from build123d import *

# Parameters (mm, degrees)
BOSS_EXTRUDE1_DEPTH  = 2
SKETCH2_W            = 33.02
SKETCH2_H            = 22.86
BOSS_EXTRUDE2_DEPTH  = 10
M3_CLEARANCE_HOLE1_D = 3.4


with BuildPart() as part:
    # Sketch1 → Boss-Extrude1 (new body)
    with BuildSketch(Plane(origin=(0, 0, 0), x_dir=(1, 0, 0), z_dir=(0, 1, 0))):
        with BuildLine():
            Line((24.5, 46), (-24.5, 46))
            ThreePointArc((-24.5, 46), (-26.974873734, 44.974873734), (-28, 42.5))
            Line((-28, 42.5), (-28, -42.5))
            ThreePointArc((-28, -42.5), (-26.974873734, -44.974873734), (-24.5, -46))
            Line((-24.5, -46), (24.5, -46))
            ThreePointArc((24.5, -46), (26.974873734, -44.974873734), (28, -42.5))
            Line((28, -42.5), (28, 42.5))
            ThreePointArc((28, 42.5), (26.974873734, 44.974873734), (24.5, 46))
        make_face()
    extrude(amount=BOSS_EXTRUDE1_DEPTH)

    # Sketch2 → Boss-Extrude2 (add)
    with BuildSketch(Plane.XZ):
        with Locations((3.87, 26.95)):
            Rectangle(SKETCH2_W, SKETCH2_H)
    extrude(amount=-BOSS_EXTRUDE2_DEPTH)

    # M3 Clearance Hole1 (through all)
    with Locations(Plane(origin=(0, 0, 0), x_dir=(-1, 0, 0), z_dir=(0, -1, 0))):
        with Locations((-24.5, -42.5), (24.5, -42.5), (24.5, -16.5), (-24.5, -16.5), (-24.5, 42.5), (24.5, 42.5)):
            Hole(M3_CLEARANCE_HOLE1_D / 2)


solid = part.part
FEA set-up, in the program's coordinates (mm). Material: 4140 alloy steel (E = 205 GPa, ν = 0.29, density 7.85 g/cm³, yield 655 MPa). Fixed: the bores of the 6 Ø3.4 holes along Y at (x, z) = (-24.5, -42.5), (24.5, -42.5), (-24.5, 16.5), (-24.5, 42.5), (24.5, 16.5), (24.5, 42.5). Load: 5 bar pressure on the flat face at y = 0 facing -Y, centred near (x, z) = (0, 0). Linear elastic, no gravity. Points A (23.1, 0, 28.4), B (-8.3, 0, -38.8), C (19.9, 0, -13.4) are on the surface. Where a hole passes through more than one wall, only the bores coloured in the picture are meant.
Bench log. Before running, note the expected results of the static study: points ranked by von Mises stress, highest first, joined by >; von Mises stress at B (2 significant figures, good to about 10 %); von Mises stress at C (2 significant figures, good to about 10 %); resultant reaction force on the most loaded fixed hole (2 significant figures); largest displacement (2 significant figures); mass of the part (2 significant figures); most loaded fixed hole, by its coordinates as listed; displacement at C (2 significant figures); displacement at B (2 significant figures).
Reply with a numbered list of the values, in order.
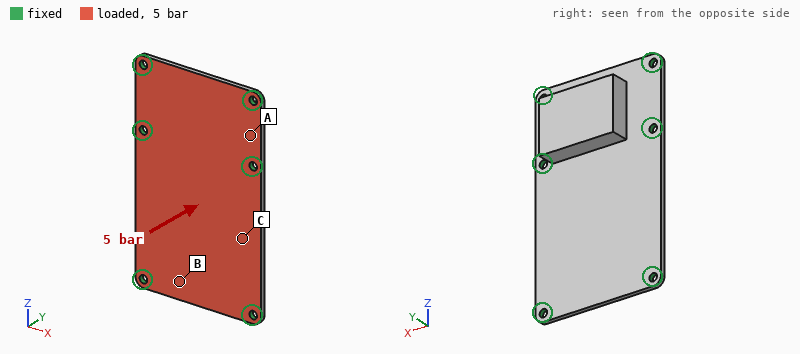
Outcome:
1. C > B > A
2. 72 MPa
3. 120 MPa
4. 930 N
5. 0.17 mm
6. 130 g
7. (24.5, 16.5)
8. 0.14 mm
9. 0.076 mm
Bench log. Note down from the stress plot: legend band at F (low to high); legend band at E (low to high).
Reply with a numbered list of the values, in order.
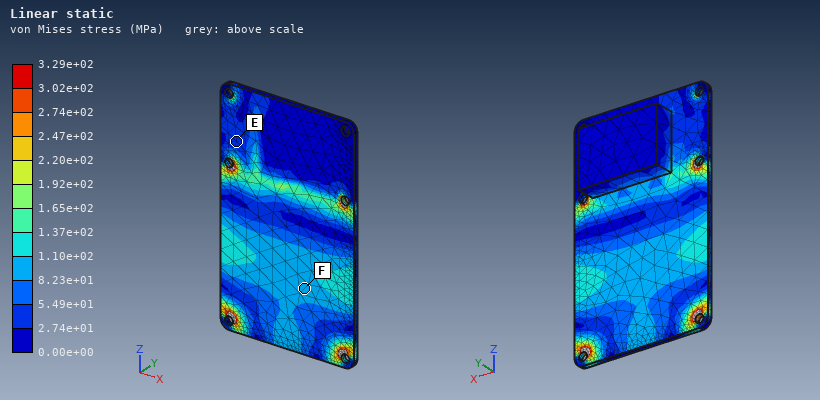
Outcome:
1. 8.23e+01 to 1.10e+02 MPa
2. 2.74e+01 to 5.49e+01 MPa
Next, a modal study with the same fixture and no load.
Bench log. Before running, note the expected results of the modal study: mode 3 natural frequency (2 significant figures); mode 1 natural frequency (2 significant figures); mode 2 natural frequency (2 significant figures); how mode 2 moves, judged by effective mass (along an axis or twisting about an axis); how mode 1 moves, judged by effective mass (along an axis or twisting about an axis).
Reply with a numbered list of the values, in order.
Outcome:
1. 4700 Hz
2. 2600 Hz
3. 3800 Hz
4. twisting about Z
5. along Y
